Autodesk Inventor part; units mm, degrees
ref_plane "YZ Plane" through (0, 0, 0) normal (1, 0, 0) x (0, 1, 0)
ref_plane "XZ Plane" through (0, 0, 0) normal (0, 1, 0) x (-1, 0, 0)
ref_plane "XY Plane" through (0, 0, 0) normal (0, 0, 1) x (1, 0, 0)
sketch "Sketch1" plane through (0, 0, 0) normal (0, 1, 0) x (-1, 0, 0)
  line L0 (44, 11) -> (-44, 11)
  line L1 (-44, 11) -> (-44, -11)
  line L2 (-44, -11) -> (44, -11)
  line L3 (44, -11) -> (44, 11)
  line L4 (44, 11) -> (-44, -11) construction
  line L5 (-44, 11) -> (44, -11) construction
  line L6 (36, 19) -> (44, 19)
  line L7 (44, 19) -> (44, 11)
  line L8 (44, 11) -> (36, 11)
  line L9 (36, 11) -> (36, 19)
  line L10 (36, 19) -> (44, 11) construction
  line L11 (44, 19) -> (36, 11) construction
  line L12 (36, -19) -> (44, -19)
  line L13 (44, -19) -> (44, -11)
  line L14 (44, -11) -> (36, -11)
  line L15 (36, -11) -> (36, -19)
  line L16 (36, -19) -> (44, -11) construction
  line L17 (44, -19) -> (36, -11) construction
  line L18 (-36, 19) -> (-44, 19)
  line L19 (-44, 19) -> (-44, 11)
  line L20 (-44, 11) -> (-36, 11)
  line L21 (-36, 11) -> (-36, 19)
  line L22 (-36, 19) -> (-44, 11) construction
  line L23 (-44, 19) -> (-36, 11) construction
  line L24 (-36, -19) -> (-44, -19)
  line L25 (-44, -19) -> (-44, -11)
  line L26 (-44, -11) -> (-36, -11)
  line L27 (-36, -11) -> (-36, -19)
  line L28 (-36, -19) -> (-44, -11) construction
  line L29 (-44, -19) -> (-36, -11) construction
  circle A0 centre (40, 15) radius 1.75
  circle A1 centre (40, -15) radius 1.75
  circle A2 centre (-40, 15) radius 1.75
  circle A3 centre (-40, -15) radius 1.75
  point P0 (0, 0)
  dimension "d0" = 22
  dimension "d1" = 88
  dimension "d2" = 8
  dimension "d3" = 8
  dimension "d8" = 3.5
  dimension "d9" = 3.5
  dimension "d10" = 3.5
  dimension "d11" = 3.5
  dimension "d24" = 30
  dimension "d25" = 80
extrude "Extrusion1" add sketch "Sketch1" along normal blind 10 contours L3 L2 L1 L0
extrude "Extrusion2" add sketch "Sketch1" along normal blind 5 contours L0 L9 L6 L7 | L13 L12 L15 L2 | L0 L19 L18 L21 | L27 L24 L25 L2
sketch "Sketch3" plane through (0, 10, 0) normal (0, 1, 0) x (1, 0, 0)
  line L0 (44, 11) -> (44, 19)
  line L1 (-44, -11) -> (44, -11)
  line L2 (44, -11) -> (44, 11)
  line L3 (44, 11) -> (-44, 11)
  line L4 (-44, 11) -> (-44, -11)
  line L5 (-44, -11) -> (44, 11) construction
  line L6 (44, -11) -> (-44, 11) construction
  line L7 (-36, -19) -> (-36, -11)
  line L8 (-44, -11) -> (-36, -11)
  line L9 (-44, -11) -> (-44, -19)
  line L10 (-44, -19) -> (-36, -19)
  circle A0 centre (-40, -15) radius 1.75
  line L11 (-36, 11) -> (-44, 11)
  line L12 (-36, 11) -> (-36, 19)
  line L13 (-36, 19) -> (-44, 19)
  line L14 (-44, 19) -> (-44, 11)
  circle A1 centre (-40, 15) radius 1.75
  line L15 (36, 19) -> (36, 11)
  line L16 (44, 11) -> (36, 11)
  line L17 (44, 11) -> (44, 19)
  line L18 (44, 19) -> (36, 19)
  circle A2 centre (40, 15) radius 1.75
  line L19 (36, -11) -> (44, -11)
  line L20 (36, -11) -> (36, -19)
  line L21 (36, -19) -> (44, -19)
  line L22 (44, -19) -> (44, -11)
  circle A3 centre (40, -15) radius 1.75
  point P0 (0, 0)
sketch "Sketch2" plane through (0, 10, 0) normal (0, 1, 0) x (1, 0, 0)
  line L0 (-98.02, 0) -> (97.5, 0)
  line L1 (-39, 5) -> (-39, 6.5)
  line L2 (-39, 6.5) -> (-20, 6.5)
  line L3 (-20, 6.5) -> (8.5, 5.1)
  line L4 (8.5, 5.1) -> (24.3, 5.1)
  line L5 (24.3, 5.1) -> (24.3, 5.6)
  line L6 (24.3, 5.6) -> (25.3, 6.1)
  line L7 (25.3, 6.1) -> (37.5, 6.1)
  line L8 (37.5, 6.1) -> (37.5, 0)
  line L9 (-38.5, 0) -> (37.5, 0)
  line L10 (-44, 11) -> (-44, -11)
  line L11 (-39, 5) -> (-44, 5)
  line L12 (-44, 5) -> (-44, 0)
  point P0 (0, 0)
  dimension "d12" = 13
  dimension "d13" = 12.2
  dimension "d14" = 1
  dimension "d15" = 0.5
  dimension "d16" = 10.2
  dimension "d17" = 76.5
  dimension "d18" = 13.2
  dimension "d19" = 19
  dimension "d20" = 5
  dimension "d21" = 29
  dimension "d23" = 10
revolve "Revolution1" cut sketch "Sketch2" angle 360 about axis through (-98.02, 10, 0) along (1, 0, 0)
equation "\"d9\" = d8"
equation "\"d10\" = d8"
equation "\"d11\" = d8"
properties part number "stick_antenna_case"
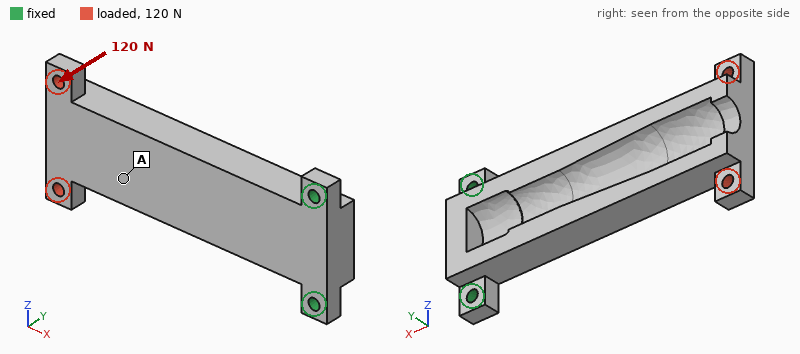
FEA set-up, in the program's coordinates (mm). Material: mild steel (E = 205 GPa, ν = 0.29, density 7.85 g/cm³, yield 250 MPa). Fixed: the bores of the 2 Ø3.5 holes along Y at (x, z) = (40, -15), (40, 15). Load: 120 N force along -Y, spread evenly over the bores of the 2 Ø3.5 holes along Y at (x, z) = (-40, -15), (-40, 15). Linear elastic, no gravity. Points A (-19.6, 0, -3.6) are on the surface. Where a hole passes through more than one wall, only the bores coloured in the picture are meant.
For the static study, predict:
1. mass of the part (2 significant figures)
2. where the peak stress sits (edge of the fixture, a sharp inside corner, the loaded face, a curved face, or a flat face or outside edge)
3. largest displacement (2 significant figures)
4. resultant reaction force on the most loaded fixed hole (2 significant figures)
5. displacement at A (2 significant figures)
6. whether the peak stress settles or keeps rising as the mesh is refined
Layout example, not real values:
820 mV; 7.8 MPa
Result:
130 g; edge of the fixture; 0.19 mm; 120 N; 0.12 mm; keeps rising
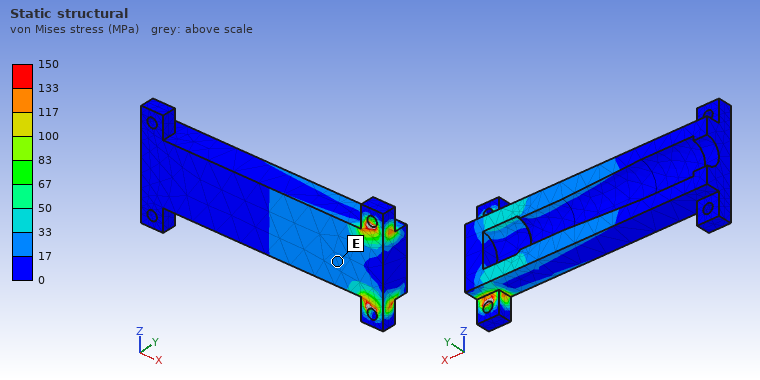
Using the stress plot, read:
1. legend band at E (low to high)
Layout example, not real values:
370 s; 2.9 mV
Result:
17 to 33 MPa
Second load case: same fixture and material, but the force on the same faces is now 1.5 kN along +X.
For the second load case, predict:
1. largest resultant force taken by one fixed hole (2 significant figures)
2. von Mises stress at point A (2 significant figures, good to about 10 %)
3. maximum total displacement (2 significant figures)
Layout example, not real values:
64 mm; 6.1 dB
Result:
790 N; 18 MPa; 39 µm
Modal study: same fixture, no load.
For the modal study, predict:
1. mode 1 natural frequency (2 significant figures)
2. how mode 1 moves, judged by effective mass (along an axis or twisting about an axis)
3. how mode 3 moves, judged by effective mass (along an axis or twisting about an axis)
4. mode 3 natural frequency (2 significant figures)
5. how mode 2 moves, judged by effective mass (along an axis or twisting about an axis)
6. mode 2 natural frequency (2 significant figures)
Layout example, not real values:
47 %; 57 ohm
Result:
660 Hz; along Y; twisting about X; 3700 Hz; along Z; 2100 Hz
